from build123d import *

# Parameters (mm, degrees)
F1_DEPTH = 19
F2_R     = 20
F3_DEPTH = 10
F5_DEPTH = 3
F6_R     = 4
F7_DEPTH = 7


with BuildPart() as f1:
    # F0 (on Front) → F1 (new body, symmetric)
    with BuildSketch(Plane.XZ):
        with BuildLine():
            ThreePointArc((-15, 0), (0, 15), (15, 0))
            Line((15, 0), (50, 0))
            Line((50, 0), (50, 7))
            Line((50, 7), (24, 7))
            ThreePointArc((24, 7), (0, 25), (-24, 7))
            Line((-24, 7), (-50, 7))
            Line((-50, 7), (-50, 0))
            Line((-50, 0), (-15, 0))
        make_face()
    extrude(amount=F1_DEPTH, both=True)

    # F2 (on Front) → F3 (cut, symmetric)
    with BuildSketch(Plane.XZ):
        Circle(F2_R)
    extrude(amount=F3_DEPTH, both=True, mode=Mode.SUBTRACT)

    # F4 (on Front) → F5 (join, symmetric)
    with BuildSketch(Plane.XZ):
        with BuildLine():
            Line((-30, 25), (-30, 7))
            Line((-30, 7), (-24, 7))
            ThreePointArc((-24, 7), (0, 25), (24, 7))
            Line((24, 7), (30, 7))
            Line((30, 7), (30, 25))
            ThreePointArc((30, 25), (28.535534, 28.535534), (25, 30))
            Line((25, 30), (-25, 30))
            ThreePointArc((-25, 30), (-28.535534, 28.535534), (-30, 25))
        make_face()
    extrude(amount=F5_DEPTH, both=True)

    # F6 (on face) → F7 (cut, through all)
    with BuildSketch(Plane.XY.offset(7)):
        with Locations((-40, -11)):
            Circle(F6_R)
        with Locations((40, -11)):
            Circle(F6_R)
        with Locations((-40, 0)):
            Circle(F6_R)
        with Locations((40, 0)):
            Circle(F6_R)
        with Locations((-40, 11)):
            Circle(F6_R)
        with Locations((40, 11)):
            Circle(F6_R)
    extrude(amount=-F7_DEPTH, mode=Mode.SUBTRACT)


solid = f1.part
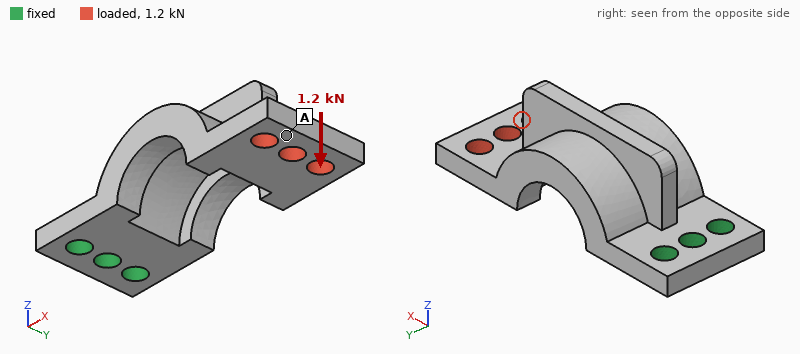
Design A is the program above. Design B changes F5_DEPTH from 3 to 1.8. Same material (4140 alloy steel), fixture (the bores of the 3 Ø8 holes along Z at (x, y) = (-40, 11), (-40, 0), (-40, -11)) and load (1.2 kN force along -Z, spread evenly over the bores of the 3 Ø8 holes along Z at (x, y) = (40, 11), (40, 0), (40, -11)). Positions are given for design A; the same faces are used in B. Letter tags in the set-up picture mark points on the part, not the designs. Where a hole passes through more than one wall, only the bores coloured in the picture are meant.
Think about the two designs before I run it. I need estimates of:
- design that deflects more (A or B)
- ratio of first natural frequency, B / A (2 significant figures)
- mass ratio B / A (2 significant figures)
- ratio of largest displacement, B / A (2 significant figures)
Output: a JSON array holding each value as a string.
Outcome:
["B", "0.99", "0.95", "1.1"]
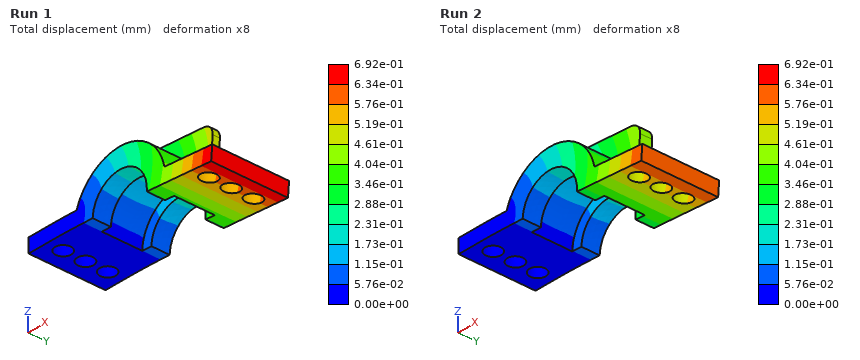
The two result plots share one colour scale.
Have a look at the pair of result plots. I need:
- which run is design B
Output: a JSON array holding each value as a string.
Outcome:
["Run 1"]
